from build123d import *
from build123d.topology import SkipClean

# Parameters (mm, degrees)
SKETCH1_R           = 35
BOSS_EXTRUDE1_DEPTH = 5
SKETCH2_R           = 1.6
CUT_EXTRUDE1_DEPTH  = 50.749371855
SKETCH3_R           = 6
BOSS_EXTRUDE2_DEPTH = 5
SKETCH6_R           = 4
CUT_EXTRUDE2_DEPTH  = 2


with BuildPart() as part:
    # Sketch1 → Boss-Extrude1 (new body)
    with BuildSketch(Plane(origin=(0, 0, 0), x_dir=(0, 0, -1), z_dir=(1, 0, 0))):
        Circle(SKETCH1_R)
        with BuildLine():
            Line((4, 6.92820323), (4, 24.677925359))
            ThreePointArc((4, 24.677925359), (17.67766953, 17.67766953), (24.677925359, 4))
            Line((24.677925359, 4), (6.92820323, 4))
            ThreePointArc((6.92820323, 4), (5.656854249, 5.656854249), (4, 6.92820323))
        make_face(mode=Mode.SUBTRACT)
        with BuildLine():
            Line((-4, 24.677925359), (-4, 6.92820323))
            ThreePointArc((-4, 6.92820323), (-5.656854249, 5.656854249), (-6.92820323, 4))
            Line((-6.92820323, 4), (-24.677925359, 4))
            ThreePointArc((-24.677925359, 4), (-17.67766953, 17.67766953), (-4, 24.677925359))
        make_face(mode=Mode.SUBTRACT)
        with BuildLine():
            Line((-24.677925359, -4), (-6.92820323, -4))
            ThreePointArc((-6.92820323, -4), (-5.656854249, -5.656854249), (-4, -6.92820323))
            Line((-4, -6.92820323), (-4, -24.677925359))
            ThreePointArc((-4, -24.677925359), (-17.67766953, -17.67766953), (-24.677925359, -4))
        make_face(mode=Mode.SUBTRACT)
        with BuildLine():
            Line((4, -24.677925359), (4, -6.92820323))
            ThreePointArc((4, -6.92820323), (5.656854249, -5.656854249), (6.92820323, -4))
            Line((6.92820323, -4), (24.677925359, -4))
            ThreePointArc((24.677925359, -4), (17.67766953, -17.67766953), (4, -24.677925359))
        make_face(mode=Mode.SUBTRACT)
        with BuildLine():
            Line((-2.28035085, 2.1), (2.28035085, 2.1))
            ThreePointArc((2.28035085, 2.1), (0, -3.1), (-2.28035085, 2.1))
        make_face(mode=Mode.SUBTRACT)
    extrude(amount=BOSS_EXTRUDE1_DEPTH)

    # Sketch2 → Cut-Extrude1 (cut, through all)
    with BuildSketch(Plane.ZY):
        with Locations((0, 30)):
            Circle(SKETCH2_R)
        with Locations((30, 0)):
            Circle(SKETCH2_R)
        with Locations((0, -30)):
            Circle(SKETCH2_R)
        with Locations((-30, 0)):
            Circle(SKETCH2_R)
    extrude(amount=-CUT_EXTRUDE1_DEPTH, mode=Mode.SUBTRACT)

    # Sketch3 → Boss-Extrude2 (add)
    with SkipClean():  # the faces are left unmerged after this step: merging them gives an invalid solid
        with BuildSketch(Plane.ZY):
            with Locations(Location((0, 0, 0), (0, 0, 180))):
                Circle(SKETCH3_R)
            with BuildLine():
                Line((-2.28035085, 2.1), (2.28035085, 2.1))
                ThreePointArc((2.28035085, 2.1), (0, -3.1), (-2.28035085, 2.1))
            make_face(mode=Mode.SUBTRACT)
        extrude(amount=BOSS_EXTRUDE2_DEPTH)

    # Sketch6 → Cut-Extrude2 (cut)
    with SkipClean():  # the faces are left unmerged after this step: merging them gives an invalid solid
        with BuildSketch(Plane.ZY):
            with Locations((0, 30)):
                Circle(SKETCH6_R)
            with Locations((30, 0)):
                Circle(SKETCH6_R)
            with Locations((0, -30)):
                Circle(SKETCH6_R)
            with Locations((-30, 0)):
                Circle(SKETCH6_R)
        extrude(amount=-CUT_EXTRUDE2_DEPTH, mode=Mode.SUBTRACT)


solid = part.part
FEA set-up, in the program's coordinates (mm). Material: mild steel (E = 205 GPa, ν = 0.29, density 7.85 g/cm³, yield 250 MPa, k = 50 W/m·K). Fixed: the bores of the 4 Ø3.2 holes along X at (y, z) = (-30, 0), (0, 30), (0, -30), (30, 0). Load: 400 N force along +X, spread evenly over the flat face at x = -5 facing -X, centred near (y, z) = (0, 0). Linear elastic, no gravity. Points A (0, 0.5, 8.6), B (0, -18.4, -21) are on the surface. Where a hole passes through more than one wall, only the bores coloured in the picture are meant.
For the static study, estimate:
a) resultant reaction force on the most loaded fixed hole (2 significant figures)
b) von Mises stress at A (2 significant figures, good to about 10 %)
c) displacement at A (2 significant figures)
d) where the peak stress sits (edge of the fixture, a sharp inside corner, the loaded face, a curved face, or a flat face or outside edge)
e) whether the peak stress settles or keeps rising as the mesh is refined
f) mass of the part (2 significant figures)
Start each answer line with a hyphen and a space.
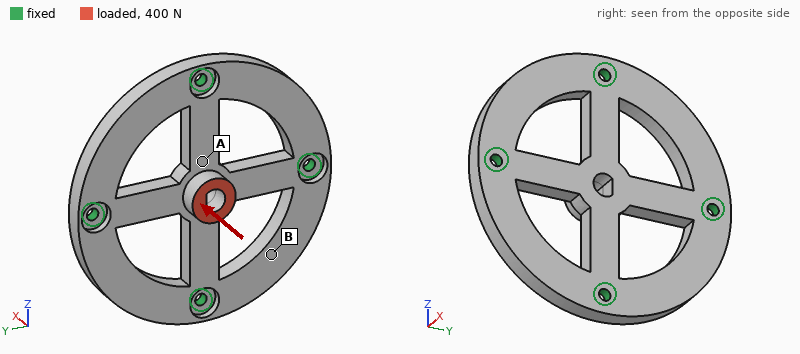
- 180 N
- 27 MPa
- 9.9 µm
- edge of the fixture
- keeps rising
- 100 g
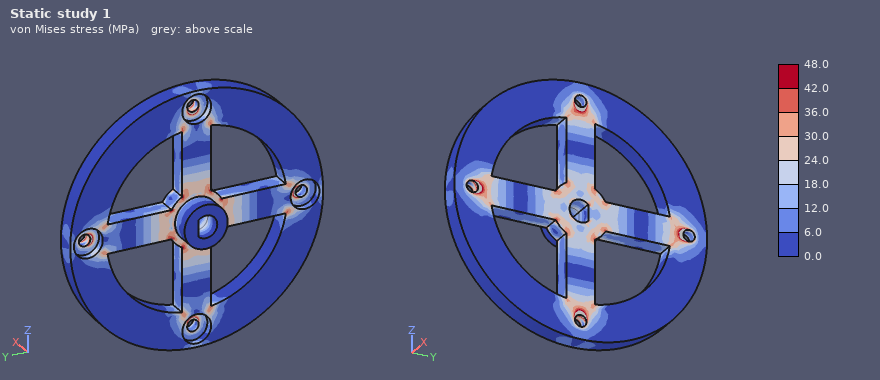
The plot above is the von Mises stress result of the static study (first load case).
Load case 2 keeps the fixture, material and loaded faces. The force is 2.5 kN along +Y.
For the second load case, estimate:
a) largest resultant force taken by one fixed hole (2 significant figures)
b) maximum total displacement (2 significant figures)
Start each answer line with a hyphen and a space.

- 1.2 kN
- 28 µm
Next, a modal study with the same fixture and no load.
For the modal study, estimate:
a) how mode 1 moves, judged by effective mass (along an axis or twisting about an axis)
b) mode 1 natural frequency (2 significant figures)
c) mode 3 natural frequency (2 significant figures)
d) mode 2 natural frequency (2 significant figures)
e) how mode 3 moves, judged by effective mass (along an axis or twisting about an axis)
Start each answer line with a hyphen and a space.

- along X
- 7000 Hz
- 8300 Hz
- 7500 Hz
- twisting about Y
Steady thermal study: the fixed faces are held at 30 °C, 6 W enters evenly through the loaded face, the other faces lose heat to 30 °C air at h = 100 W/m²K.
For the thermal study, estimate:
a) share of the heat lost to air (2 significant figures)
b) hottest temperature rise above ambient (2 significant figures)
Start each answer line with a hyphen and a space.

- 45 %
- 21 K
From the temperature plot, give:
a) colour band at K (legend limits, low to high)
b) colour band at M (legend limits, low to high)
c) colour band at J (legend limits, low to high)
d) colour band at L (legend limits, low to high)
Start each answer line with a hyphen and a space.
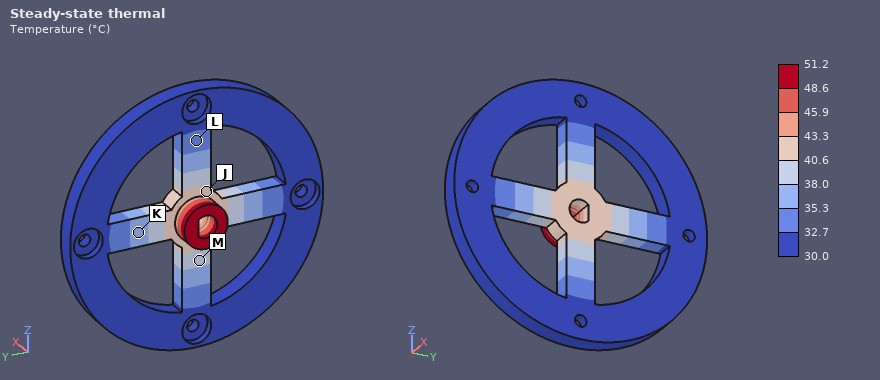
- 35.3 to 38.0 °C
- 38.0 to 40.6 °C
- 40.6 to 43.3 °C
- 32.7 to 35.3 °C
